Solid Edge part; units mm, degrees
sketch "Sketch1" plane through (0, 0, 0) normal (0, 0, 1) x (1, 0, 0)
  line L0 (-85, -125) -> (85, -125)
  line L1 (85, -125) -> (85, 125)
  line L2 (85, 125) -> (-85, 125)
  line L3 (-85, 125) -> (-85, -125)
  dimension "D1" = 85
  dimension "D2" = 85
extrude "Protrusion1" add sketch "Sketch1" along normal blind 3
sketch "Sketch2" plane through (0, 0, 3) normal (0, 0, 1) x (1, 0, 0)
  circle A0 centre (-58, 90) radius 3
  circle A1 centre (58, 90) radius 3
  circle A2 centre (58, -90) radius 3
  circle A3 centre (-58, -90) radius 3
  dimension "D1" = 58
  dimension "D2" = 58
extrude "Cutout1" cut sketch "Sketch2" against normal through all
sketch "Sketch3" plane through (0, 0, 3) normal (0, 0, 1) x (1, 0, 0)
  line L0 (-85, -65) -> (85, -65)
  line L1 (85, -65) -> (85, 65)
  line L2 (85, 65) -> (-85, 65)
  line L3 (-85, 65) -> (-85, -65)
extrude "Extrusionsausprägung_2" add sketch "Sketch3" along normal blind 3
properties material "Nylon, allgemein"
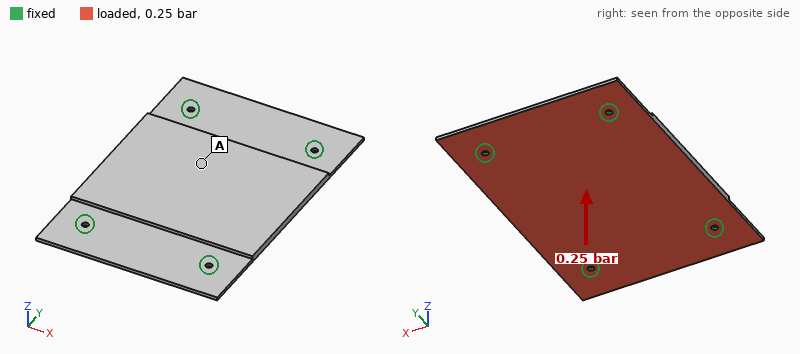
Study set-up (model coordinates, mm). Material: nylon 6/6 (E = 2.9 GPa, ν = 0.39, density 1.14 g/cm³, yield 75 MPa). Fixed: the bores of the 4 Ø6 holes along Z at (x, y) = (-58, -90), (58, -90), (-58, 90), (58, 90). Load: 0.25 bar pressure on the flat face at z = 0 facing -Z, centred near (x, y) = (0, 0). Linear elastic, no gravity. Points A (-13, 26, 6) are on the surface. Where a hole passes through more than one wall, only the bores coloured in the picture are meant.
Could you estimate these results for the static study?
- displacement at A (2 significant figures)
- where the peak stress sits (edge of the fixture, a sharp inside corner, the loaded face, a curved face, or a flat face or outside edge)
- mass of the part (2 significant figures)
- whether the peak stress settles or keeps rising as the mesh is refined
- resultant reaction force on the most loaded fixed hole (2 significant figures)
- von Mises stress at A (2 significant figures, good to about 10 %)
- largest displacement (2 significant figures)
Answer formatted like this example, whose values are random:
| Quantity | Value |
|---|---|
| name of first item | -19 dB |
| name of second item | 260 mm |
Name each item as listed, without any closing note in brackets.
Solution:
| Quantity | Value |
|---|---|
| displacement at A | 3.2 mm |
| where the peak stress sits | edge of the fixture |
| mass of the part | 220 g |
| whether the peak stress settles or keeps rising as the mesh is refined | keeps rising |
| resultant reaction force on the most loaded fixed hole | 590 N |
| von Mises stress at A | 7.0 MPa |
| largest displacement | 3.5 mm |
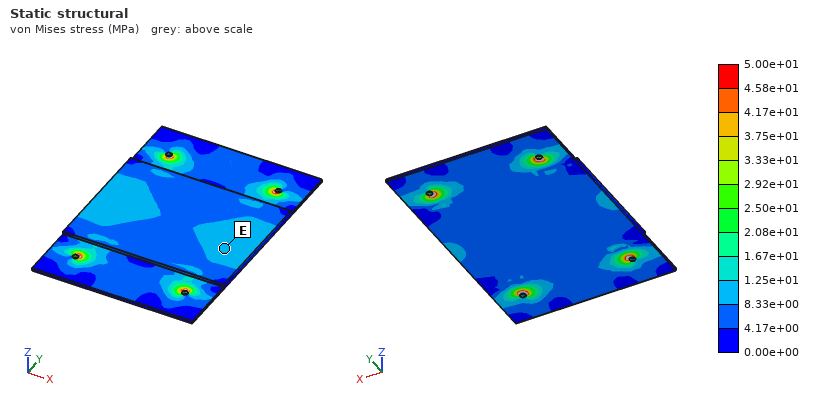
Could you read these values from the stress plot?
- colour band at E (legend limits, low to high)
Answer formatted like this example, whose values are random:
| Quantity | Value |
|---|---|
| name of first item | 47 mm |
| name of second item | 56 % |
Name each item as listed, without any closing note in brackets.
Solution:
| Quantity | Value |
|---|---|
| colour band at E | 8.33e+00 to 1.25e+01 MPa |
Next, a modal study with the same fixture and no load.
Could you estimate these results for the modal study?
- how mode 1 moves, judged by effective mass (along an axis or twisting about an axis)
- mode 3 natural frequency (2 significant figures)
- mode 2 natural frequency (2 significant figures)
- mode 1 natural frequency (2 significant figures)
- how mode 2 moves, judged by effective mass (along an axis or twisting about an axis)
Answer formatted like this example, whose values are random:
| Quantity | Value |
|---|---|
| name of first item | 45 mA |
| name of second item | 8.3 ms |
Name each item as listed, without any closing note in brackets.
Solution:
| Quantity | Value |
|---|---|
| how mode 1 moves, judged by effective mass | along Z |
| mode 3 natural frequency | 340 Hz |
| mode 2 natural frequency | 240 Hz |
| mode 1 natural frequency | 180 Hz |
| how mode 2 moves, judged by effective mass | twisting about Y |
